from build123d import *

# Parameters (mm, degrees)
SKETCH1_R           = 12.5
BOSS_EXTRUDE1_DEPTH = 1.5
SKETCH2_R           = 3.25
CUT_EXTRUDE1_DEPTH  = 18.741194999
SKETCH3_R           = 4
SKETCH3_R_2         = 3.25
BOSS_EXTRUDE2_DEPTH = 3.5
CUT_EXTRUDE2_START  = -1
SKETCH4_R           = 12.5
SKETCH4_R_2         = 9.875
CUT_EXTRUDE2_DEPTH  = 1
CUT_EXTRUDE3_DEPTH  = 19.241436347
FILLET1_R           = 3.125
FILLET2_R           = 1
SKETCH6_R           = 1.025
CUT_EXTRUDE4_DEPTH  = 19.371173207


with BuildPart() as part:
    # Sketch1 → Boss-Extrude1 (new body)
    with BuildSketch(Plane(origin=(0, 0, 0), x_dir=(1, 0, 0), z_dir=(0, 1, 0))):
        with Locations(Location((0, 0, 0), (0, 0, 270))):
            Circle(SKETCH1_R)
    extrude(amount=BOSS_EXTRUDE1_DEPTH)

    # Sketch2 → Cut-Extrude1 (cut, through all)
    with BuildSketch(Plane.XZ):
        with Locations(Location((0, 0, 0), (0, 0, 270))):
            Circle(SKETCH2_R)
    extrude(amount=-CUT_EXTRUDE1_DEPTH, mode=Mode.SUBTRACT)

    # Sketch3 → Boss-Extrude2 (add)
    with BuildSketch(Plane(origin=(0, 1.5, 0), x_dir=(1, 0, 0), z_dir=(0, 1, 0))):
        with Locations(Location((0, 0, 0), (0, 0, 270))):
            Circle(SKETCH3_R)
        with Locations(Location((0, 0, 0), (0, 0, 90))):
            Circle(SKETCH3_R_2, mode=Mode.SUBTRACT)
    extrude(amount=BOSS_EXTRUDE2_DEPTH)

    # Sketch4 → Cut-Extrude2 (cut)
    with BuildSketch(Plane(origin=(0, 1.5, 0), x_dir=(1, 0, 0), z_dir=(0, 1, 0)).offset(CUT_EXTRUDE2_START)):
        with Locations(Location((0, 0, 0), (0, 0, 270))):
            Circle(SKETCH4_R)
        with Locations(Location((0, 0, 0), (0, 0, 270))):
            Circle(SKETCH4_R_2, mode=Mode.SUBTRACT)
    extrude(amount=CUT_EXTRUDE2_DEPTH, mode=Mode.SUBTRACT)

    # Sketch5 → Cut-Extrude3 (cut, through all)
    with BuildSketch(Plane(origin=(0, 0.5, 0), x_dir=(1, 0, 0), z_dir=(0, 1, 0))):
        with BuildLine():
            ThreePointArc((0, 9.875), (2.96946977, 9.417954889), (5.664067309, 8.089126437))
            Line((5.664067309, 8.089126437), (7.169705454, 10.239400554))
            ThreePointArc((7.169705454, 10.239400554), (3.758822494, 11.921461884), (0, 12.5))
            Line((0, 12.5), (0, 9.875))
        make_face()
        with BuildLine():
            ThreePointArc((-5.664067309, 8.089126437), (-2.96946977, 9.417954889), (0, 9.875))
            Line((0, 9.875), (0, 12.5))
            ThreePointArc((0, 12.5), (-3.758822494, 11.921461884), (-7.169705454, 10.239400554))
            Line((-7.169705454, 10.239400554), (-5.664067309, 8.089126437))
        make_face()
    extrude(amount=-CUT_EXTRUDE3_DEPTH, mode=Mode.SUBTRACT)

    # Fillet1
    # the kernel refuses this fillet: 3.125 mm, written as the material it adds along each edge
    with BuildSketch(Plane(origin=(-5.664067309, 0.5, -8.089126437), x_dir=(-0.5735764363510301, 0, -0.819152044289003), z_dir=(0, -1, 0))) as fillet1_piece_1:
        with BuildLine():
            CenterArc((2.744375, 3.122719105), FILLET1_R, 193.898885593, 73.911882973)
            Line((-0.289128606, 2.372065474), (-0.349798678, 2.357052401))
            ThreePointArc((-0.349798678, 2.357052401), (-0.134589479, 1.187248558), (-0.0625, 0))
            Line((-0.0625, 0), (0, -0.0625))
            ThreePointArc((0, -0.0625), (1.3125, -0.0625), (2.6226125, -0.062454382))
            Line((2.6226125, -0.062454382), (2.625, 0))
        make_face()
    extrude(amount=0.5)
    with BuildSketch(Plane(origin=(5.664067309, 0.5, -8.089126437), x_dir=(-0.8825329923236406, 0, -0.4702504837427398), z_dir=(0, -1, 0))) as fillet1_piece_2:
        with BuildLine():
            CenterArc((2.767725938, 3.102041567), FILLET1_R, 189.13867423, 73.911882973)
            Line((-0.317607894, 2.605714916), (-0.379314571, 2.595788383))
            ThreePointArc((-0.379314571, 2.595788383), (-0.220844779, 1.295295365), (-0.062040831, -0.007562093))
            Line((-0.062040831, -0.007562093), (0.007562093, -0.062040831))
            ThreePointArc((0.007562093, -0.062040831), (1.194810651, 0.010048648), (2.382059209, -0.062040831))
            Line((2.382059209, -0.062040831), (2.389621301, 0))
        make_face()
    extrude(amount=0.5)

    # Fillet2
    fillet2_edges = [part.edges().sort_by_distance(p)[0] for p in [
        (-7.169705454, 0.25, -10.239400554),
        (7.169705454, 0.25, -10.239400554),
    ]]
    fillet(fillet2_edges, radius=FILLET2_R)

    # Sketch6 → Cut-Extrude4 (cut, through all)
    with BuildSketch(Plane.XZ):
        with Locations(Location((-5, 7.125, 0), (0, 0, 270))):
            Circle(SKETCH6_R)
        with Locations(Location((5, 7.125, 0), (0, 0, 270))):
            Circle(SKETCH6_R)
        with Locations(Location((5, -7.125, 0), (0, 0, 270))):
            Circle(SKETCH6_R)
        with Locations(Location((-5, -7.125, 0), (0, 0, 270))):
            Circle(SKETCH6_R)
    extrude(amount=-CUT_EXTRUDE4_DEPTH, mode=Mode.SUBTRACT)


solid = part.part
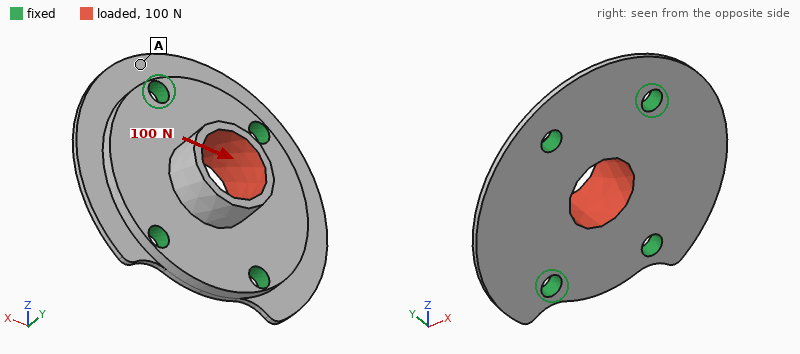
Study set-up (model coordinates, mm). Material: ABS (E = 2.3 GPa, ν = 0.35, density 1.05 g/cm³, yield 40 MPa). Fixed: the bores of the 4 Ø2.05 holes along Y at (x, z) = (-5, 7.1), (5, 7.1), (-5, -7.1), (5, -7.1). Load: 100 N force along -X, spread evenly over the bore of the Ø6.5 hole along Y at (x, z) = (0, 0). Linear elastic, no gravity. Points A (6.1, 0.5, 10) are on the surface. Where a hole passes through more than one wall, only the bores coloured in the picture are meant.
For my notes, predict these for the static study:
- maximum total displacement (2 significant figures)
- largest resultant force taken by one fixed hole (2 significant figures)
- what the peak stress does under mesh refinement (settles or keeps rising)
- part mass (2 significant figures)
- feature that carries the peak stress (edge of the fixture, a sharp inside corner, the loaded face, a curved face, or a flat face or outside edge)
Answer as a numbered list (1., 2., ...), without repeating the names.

1. 83 µm
2. 28 N
3. keeps rising
4. 0.55 g
5. edge of the fixture
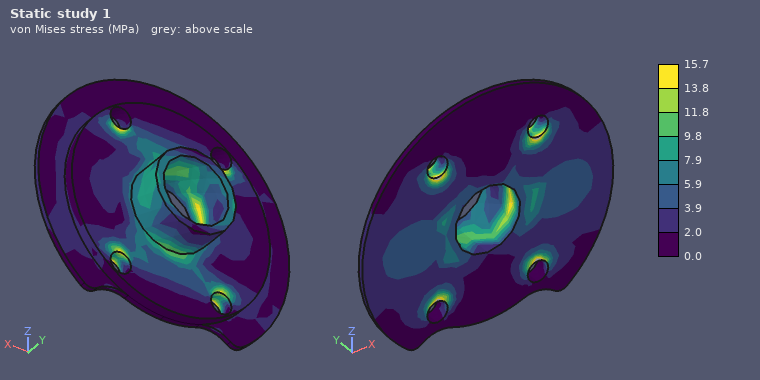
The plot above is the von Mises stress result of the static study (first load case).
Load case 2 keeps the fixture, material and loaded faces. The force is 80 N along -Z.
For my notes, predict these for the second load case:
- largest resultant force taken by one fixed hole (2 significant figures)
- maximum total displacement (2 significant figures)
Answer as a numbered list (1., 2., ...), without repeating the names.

1. 22 N
2. 51 µm
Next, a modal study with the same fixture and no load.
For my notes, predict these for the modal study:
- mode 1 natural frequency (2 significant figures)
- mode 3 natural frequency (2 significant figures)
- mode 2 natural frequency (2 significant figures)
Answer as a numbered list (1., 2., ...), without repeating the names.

1. 7400 Hz
2. 12 kHz
3. 7500 Hz
